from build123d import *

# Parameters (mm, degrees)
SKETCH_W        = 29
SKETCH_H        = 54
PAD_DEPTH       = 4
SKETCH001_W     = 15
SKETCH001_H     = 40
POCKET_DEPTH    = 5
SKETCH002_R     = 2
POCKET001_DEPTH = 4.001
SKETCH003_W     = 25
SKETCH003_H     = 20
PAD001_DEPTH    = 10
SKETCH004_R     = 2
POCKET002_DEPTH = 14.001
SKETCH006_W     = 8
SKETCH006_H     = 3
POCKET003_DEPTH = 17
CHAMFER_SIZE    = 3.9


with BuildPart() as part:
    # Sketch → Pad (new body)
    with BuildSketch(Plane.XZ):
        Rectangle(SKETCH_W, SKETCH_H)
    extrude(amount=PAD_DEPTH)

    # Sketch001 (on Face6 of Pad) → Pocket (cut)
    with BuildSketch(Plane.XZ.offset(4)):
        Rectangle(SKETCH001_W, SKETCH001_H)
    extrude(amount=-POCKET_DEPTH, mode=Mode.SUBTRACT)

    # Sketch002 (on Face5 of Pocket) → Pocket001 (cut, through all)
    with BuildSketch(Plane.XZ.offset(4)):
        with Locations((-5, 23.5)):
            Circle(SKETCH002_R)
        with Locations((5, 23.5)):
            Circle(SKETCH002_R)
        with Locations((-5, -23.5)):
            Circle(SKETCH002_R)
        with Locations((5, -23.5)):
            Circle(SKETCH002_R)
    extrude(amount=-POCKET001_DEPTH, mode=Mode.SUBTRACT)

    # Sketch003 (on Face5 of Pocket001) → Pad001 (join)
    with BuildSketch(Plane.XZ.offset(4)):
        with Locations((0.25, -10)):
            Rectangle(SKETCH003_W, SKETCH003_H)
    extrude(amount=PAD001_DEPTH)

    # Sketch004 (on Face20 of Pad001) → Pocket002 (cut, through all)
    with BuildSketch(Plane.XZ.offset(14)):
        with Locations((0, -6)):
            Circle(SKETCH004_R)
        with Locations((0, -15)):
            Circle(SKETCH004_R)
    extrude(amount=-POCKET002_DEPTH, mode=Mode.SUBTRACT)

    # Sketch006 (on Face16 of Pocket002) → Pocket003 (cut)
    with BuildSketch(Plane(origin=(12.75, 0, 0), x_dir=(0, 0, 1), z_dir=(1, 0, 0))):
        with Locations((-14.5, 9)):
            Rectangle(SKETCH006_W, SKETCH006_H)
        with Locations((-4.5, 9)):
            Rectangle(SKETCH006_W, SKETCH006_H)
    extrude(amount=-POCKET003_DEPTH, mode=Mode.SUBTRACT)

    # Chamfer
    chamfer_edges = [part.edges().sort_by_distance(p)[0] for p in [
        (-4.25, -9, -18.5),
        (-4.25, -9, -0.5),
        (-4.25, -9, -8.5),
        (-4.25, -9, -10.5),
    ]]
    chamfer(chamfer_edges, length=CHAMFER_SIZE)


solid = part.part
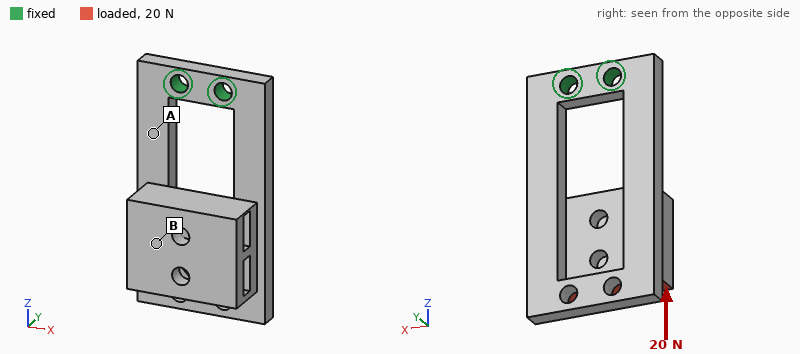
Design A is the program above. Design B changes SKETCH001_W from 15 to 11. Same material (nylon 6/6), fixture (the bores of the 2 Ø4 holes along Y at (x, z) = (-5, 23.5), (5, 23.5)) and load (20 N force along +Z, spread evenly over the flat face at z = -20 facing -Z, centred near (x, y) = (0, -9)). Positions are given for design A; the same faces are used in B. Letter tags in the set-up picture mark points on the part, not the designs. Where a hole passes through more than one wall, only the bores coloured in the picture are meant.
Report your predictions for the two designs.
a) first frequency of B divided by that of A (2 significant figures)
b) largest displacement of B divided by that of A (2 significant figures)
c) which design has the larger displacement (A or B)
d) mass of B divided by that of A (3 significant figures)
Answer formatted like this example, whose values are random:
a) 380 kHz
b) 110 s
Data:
a) 1.2
b) 0.74
c) A
d) 1.08
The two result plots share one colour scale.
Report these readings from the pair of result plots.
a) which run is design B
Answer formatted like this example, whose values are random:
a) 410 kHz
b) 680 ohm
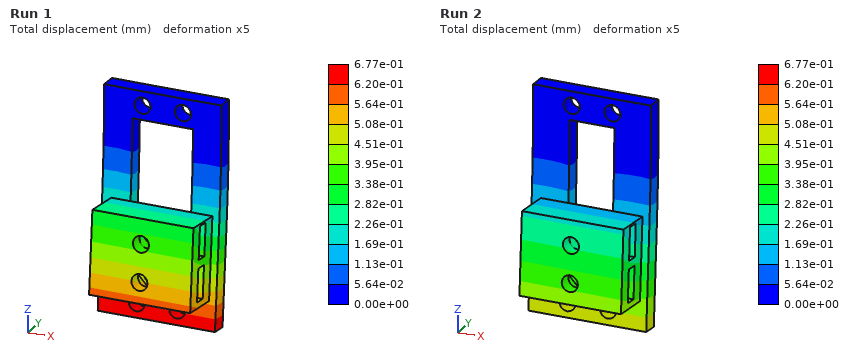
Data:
a) Run 2
